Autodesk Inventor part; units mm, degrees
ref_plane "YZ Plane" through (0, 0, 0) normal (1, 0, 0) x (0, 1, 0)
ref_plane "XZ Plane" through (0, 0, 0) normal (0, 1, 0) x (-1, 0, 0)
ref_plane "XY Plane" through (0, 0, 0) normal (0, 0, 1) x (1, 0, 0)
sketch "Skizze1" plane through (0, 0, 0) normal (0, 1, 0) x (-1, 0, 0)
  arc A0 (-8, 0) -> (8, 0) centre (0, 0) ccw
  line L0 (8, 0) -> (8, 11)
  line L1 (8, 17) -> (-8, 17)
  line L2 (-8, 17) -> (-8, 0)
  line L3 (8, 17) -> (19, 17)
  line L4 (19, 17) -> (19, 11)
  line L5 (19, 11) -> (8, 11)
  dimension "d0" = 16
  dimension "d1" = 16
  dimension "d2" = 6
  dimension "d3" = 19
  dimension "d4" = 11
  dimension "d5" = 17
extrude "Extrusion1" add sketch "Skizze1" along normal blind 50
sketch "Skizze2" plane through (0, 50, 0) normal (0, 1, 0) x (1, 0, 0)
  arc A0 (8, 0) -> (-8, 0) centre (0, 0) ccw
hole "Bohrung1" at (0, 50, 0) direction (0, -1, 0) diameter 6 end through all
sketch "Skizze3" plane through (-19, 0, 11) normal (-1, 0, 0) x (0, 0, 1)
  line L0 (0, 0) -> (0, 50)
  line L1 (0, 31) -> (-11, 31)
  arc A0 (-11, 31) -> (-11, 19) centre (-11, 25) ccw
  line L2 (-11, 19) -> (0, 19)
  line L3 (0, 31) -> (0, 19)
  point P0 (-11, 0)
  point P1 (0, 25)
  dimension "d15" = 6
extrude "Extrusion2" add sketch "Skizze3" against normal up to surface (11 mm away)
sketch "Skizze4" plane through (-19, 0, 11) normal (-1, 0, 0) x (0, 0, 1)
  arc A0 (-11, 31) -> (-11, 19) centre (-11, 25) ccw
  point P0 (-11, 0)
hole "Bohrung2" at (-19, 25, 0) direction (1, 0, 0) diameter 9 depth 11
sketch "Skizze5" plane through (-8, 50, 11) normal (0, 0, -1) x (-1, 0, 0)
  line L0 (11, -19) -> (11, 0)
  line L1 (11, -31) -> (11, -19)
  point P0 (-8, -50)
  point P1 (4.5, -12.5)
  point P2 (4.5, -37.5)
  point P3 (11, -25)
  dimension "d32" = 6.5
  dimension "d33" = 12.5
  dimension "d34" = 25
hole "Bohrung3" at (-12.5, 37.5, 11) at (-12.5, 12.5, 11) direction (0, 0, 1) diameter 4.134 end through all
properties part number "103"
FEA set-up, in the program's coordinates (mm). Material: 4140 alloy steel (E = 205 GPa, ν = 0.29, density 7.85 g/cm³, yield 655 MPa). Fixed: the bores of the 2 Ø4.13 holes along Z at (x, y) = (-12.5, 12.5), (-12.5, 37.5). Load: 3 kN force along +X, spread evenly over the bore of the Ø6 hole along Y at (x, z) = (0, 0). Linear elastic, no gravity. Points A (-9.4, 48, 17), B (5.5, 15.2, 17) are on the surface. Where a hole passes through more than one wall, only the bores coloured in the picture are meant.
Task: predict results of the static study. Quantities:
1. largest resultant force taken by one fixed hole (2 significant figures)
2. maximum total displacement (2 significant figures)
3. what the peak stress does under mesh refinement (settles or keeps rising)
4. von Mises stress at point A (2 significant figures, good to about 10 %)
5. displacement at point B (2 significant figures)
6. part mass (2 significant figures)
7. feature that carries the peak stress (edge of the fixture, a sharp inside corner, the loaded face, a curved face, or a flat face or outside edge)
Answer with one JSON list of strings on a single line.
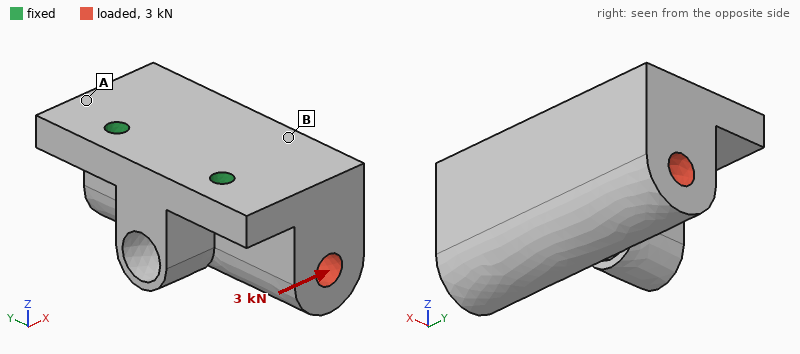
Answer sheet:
["1.5 kN", "39 µm", "keeps rising", "53 MPa", "24 µm", "170 g", "edge of the fixture"]
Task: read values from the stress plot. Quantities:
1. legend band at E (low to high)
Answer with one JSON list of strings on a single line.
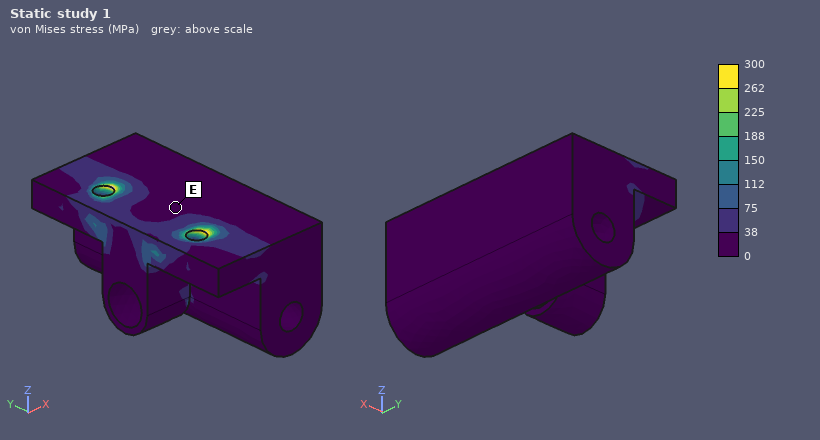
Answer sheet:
["0 to 38 MPa"]
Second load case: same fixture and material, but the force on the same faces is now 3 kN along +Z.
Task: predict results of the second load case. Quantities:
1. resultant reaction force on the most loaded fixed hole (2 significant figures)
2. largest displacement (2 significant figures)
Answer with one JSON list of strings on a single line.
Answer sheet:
["1.5 kN", "29 µm"]
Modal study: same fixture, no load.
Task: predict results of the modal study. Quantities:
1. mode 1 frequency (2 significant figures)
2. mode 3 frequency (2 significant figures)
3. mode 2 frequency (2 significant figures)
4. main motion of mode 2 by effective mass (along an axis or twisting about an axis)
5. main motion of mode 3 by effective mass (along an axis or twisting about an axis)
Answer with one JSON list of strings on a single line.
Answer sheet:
["4500 Hz", "13 kHz", "10 kHz", "along Y", "along Y"]
